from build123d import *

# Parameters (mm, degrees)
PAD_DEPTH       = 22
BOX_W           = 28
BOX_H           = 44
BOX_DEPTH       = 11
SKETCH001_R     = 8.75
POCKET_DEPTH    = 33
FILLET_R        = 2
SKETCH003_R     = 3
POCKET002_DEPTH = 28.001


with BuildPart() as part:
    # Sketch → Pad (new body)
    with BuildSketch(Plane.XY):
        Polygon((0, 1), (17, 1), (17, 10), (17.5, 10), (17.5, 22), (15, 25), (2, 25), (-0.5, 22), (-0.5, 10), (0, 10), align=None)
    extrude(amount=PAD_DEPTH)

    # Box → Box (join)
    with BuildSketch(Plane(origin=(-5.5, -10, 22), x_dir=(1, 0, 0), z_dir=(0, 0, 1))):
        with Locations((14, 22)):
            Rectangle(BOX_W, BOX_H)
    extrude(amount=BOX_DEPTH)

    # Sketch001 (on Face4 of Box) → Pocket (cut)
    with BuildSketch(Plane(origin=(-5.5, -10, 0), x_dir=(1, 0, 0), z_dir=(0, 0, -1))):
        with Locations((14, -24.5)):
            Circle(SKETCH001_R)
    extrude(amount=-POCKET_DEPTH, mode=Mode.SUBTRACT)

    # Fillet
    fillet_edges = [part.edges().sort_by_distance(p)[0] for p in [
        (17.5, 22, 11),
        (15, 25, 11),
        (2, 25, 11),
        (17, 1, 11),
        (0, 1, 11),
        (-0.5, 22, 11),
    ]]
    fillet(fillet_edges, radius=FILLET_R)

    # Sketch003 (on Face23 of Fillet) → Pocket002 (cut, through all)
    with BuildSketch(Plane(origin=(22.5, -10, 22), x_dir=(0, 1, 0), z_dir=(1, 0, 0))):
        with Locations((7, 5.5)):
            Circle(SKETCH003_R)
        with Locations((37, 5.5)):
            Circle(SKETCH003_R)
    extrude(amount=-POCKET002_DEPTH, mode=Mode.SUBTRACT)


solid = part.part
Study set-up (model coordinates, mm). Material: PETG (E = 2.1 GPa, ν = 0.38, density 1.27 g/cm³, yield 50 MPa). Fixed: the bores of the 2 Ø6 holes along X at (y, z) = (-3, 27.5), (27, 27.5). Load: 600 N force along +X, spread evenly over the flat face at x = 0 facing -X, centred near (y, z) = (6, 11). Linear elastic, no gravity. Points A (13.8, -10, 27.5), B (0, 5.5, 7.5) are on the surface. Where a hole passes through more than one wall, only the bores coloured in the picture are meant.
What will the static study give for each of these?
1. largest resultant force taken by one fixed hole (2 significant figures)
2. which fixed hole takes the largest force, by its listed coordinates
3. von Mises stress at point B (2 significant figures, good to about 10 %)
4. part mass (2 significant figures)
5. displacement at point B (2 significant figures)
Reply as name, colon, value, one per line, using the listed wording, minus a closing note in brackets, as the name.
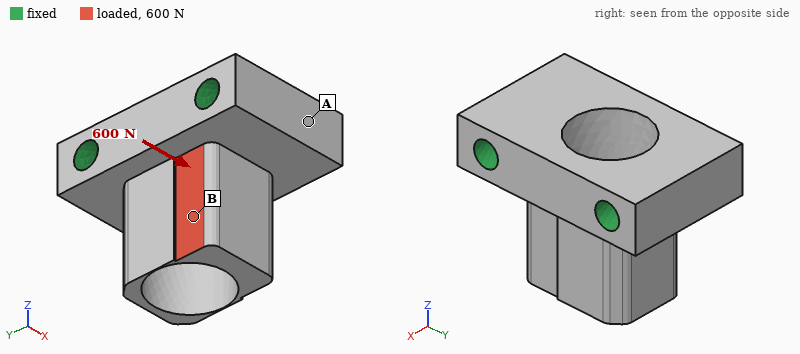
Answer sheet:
largest resultant force taken by one fixed hole: 540 N
which fixed hole takes the largest force, by its listed coordinates: (-3, 27.5)
von Mises stress at point B: 7.1 MPa
part mass: 17 g
displacement at point B: 0.37 mm
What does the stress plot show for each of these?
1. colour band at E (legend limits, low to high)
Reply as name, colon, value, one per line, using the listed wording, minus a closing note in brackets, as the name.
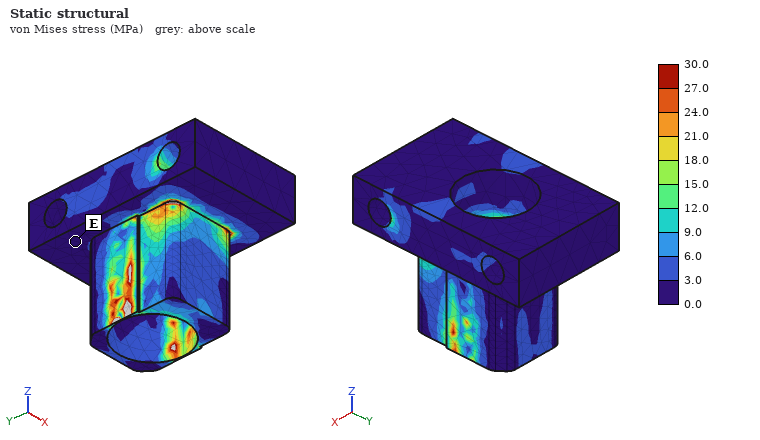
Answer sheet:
colour band at E: 0.0 to 3.0 MPa
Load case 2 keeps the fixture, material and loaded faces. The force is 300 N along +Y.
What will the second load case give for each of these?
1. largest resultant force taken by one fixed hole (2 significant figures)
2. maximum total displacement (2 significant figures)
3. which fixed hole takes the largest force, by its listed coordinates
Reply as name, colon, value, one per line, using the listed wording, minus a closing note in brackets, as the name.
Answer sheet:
largest resultant force taken by one fixed hole: 250 N
maximum total displacement: 0.33 mm
which fixed hole takes the largest force, by its listed coordinates: (-3, 27.5)
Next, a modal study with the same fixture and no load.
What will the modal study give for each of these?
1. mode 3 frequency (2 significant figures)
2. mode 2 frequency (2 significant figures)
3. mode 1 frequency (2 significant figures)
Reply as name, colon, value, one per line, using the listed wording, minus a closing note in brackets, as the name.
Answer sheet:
mode 3 frequency: 4300 Hz
mode 2 frequency: 4100 Hz
mode 1 frequency: 4000 Hz
